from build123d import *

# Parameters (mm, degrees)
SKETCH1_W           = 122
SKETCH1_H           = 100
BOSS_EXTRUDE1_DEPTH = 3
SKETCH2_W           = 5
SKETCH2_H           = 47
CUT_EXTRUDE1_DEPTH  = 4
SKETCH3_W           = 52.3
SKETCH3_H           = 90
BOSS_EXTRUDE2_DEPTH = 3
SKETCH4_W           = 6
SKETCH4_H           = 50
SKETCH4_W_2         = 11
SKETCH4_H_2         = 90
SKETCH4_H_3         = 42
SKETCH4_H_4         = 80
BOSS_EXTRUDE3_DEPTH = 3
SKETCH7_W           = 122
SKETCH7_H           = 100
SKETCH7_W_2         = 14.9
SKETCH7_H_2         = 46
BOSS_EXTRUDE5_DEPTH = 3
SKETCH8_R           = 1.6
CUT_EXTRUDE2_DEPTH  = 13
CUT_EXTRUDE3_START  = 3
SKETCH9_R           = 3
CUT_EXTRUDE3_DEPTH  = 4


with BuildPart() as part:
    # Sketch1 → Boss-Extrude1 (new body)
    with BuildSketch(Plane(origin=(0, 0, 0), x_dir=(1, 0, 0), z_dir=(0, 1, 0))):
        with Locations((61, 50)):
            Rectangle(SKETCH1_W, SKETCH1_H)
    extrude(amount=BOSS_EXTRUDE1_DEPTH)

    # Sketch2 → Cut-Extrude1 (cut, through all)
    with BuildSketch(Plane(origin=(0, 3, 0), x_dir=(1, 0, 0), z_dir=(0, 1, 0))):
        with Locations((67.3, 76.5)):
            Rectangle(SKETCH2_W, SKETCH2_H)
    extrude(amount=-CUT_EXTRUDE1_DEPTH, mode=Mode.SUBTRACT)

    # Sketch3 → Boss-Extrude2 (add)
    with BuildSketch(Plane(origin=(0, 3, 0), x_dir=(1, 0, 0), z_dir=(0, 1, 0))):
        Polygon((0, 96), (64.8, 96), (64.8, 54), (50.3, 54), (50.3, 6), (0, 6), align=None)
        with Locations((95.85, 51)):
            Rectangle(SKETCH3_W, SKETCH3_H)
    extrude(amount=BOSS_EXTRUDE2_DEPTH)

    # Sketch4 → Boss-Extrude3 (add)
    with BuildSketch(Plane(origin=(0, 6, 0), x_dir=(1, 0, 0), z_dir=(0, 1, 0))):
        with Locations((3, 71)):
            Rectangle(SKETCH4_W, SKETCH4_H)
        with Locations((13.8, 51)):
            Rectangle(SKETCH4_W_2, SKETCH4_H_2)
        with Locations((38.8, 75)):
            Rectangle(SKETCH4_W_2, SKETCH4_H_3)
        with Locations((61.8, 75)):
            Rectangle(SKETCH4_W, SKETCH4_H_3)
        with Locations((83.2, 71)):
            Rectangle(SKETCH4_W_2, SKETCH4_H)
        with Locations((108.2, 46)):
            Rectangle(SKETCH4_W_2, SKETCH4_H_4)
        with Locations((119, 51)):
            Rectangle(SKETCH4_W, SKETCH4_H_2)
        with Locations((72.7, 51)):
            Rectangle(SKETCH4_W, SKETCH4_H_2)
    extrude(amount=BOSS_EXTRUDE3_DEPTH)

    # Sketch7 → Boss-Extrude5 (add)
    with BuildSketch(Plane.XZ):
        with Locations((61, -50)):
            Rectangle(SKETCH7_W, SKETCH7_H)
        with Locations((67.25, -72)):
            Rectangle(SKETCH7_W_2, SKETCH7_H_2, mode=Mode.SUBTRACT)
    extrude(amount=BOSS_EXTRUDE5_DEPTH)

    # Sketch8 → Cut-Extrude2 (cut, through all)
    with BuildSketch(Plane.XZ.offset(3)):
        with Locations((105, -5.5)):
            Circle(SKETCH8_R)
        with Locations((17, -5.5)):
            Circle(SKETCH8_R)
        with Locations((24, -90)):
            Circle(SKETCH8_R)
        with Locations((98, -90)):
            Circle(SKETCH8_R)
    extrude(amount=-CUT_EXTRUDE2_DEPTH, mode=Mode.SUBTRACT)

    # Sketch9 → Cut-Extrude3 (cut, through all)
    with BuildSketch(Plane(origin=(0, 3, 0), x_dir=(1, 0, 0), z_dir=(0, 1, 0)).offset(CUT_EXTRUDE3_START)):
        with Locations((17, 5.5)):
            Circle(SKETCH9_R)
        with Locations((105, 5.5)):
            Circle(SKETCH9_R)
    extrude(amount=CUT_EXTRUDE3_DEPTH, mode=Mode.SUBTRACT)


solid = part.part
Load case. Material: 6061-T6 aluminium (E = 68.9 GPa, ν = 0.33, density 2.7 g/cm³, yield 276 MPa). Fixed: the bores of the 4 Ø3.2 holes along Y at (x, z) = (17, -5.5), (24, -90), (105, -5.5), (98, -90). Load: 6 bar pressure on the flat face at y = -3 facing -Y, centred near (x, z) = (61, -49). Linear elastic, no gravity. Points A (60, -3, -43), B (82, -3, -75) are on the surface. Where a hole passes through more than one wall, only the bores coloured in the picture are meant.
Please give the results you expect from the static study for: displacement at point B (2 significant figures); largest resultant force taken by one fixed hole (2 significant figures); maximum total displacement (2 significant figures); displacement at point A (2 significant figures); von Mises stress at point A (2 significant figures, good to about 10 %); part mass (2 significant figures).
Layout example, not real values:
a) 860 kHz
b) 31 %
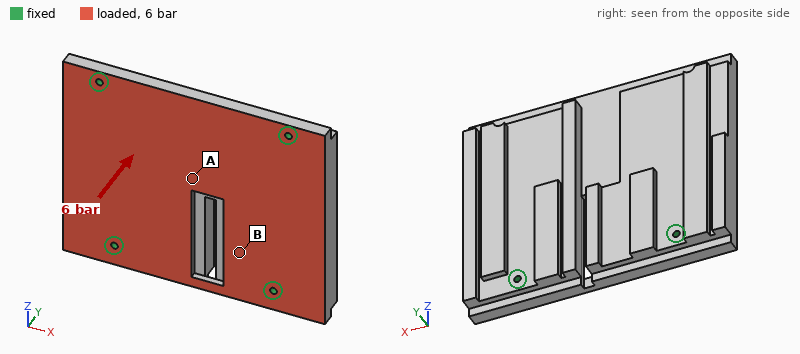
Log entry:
a) 35 µm
b) 1.9 kN
c) 83 µm
d) 80 µm
e) 28 MPa
f) 310 g
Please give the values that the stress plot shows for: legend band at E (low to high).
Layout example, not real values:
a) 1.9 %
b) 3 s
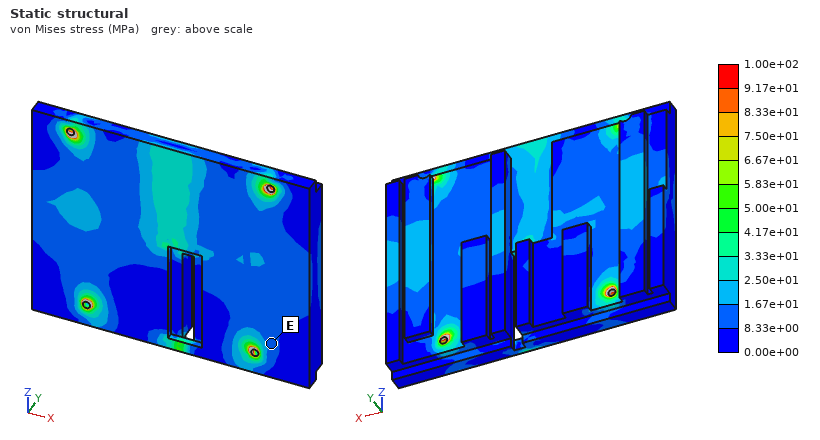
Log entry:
a) 8.33e+00 to 1.67e+01 MPa
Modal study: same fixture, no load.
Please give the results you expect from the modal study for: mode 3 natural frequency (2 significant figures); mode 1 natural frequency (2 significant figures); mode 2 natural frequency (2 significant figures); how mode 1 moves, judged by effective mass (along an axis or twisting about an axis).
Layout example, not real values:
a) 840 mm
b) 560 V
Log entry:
a) 4900 Hz
b) 3200 Hz
c) 4800 Hz
d) along Y
